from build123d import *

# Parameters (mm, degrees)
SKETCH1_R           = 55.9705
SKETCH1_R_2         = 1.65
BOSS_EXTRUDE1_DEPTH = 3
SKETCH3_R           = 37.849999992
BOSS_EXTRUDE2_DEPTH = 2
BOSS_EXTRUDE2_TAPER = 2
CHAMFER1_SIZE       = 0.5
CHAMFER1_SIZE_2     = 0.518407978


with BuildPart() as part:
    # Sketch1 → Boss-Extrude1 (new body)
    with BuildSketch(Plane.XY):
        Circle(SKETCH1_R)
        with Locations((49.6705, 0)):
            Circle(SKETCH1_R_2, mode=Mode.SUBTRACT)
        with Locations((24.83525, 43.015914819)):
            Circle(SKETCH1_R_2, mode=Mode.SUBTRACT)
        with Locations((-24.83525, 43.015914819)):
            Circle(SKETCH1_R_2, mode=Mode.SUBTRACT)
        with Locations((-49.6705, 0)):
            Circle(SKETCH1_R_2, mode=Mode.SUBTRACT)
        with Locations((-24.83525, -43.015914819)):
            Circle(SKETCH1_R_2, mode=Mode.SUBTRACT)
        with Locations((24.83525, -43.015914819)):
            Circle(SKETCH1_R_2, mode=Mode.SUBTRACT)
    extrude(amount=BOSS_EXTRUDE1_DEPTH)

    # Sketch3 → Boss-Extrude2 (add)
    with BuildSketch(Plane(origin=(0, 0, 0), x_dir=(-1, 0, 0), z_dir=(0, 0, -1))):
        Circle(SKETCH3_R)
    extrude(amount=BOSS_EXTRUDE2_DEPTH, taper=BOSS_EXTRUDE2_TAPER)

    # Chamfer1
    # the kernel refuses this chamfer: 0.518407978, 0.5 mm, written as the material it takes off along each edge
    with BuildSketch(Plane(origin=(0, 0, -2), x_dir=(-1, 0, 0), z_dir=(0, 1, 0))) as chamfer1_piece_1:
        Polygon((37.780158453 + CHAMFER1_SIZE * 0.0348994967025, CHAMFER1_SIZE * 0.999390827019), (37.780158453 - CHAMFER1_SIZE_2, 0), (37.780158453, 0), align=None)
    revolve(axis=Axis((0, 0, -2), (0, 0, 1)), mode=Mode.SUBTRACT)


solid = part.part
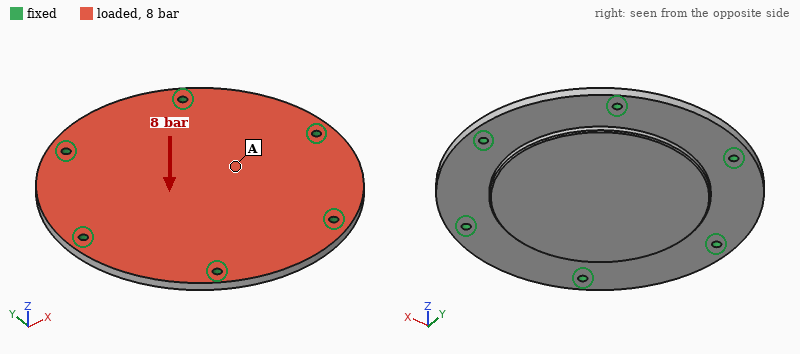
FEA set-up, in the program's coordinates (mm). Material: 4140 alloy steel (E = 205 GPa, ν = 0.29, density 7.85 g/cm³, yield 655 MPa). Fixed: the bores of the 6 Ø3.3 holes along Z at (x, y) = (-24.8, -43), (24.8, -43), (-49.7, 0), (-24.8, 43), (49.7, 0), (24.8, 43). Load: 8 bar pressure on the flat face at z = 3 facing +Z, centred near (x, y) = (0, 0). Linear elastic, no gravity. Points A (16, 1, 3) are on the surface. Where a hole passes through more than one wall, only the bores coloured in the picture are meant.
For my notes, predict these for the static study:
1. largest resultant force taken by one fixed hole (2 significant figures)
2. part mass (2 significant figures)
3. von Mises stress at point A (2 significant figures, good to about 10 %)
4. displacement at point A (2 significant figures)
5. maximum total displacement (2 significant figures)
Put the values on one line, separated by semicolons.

1.6 kN; 300 g; 46 MPa; 77 µm; 87 µm
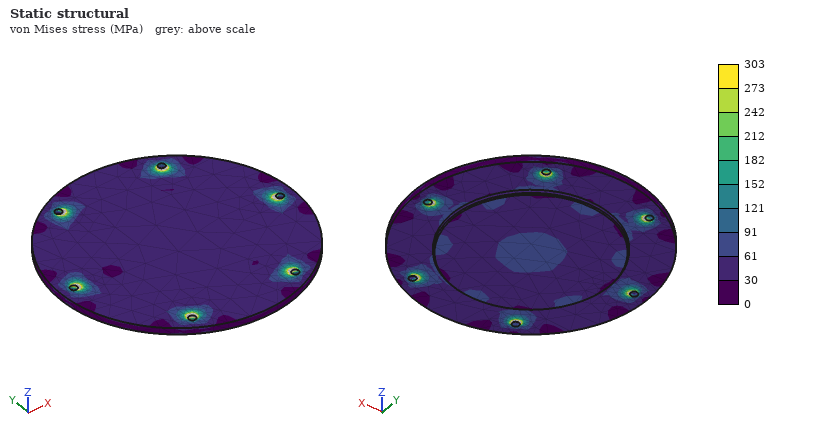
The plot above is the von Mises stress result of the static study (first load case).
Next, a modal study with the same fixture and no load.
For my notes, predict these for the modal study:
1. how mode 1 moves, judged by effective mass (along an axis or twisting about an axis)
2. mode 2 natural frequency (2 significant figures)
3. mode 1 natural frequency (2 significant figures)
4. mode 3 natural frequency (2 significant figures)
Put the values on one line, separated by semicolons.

along Z; 5700 Hz; 3000 Hz; 5700 Hz
